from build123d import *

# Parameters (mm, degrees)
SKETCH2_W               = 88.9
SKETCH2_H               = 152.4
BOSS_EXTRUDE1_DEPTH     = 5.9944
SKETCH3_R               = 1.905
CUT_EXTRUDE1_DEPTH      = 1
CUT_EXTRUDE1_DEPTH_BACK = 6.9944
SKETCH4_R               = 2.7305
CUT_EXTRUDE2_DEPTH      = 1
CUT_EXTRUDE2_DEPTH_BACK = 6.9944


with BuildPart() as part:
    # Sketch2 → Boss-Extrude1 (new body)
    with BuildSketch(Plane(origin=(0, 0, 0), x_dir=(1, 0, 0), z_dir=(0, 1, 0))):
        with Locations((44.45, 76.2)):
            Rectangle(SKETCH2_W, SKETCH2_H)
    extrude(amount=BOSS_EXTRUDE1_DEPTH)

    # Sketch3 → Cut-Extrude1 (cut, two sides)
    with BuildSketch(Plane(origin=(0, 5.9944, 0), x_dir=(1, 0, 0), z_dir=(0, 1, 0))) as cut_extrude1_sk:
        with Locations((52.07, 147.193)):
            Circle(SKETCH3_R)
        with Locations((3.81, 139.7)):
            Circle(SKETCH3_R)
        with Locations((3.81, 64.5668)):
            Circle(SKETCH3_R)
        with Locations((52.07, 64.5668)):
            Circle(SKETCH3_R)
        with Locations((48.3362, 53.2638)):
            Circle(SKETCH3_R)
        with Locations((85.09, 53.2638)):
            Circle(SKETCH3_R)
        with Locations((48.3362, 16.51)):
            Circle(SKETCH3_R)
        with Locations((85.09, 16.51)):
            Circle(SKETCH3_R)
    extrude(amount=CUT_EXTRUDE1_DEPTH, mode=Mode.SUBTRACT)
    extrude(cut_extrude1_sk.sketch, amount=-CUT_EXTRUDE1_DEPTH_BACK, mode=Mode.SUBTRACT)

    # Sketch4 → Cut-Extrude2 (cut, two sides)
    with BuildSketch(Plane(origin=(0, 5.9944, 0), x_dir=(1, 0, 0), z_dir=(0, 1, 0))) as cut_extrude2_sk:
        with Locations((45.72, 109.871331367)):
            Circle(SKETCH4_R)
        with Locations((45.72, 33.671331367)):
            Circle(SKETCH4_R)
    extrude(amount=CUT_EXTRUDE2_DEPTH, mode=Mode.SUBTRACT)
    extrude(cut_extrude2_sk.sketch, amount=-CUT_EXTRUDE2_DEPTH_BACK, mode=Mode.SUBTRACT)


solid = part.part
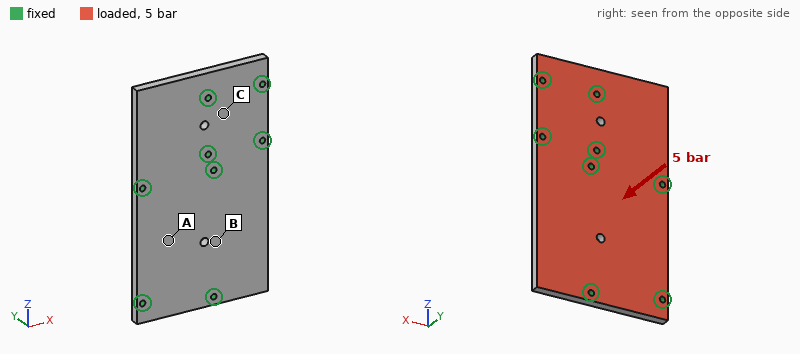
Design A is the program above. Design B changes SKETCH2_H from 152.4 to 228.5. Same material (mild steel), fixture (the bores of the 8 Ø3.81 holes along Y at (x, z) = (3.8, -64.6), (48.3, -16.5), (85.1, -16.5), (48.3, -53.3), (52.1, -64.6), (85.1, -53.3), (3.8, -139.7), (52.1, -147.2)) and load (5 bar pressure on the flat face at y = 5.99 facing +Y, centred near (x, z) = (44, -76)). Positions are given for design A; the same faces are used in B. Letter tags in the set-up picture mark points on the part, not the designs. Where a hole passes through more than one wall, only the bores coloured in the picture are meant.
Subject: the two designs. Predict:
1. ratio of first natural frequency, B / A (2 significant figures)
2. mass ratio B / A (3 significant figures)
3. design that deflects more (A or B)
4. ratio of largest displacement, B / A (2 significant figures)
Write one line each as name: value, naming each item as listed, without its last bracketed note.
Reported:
ratio of first natural frequency, B / A: 0.46
mass ratio B / A: 1.50
design that deflects more: B
ratio of largest displacement, B / A: 5.4
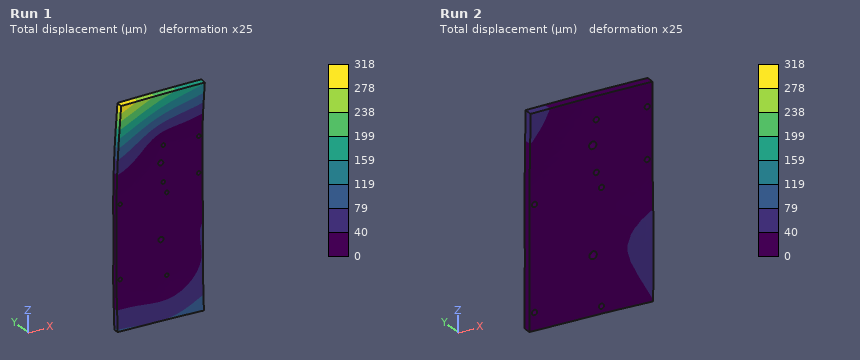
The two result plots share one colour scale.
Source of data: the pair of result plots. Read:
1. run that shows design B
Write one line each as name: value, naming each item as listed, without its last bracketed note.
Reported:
run that shows design B: Run 1
